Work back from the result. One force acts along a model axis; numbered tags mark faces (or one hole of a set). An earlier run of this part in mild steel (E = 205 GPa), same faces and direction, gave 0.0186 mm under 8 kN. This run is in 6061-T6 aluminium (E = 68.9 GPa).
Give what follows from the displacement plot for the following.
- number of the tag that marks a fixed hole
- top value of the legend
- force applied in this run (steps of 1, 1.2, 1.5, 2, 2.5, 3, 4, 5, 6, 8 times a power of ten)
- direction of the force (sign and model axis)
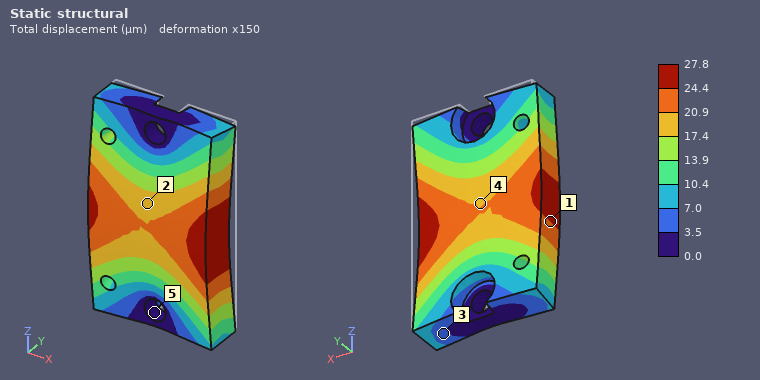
5
27.8 µm
4 kN
-Y
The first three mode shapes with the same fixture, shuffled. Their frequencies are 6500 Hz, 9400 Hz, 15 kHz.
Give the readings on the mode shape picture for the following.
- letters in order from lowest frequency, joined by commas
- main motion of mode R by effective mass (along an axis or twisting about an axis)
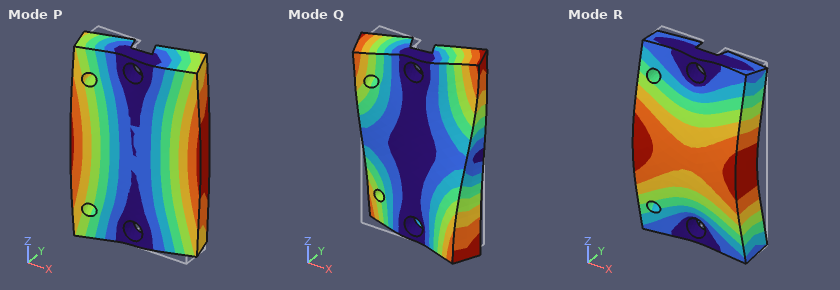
P, R, Q
along Y
